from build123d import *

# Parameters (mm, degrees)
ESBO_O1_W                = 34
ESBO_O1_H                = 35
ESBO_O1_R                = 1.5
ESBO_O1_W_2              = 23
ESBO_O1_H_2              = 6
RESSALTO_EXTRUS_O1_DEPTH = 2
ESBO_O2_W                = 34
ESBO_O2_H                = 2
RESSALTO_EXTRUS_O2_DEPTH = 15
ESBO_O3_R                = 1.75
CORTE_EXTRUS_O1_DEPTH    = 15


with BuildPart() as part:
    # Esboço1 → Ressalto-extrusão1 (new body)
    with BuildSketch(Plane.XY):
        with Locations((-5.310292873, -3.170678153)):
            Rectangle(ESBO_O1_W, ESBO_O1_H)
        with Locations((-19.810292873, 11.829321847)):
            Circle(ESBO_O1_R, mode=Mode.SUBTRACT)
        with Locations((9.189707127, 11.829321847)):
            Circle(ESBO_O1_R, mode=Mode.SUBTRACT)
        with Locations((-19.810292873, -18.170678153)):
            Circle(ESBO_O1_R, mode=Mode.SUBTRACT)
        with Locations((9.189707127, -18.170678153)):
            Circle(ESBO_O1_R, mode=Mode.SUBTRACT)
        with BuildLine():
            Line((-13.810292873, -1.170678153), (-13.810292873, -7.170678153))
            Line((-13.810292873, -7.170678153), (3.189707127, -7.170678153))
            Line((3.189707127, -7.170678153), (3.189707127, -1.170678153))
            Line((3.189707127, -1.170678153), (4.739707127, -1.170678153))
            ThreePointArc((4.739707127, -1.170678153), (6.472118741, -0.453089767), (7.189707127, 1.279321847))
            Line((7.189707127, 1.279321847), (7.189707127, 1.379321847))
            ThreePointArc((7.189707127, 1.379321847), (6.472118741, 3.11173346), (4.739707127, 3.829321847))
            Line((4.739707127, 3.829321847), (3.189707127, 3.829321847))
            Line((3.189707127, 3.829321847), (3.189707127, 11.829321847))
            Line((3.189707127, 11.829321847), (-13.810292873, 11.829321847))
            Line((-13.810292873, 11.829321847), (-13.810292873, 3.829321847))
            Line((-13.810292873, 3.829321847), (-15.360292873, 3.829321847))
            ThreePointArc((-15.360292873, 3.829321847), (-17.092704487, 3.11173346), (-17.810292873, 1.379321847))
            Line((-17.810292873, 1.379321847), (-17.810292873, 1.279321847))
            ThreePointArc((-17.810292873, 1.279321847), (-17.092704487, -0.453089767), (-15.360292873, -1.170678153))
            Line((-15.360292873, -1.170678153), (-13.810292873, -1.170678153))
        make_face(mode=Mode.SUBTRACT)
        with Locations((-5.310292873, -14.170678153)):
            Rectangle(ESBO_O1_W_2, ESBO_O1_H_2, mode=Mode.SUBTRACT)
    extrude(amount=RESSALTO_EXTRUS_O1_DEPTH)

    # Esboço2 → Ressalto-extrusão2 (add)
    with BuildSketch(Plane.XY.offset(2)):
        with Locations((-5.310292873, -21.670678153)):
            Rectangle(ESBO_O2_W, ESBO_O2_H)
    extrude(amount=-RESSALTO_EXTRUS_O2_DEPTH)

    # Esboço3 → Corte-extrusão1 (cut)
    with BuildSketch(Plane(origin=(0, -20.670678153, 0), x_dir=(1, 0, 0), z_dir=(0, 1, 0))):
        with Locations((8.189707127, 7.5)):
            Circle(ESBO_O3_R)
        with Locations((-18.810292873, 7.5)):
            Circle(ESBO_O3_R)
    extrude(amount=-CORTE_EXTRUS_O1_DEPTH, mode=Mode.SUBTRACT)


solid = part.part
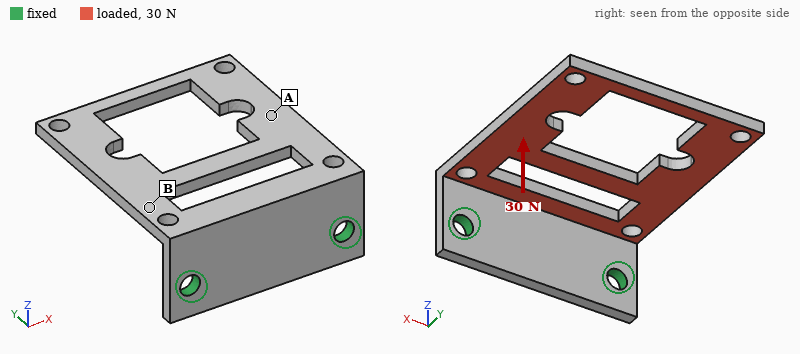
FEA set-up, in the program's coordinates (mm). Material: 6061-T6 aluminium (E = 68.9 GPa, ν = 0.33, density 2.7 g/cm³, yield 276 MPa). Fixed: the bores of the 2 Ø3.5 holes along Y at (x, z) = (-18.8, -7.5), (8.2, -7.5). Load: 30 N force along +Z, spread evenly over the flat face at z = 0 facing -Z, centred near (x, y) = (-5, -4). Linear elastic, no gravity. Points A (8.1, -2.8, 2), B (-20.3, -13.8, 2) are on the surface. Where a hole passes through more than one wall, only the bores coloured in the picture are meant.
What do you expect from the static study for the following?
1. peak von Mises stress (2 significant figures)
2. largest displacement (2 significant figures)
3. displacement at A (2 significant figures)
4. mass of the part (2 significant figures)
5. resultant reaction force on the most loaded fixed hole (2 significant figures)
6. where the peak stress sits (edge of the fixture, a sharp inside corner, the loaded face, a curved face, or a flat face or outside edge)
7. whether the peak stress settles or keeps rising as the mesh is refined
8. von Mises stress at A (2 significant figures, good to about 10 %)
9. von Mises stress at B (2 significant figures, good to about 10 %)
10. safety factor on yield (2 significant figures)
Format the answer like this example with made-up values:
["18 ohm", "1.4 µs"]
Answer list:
["140 MPa", "0.48 mm", "0.20 mm", "6.2 g", "15 N", "the loaded face", "settles", "14 MPa", "42 MPa", "1.9"]
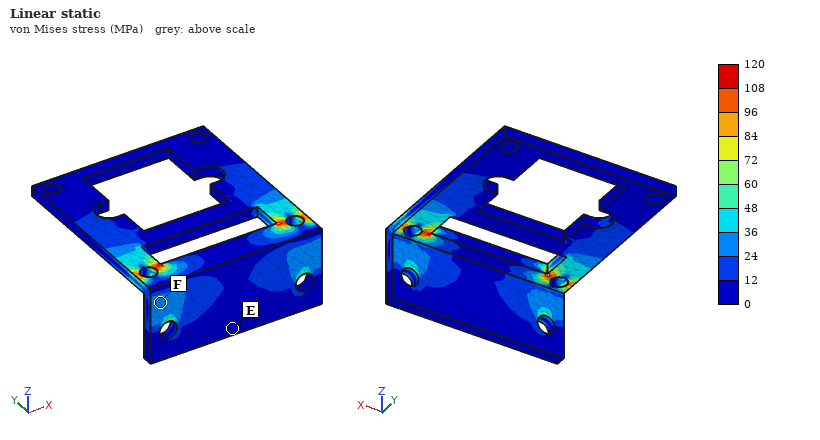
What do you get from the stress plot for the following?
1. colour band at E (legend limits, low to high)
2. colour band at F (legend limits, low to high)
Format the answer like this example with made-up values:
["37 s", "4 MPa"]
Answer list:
["0 to 12 MPa", "24 to 36 MPa"]
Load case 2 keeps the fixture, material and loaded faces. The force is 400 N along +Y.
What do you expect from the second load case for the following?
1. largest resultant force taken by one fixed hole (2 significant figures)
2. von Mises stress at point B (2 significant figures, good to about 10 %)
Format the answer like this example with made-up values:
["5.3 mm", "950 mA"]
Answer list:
["200 N", "32 MPa"]
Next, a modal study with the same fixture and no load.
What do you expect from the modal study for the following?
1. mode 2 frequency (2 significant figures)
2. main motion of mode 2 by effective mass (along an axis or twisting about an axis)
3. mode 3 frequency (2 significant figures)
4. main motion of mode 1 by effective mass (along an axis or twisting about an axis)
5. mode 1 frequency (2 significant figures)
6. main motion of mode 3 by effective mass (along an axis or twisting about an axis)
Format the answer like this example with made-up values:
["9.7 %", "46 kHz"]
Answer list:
["2100 Hz", "twisting about Y", "3600 Hz", "along Z", "810 Hz", "along X"]
